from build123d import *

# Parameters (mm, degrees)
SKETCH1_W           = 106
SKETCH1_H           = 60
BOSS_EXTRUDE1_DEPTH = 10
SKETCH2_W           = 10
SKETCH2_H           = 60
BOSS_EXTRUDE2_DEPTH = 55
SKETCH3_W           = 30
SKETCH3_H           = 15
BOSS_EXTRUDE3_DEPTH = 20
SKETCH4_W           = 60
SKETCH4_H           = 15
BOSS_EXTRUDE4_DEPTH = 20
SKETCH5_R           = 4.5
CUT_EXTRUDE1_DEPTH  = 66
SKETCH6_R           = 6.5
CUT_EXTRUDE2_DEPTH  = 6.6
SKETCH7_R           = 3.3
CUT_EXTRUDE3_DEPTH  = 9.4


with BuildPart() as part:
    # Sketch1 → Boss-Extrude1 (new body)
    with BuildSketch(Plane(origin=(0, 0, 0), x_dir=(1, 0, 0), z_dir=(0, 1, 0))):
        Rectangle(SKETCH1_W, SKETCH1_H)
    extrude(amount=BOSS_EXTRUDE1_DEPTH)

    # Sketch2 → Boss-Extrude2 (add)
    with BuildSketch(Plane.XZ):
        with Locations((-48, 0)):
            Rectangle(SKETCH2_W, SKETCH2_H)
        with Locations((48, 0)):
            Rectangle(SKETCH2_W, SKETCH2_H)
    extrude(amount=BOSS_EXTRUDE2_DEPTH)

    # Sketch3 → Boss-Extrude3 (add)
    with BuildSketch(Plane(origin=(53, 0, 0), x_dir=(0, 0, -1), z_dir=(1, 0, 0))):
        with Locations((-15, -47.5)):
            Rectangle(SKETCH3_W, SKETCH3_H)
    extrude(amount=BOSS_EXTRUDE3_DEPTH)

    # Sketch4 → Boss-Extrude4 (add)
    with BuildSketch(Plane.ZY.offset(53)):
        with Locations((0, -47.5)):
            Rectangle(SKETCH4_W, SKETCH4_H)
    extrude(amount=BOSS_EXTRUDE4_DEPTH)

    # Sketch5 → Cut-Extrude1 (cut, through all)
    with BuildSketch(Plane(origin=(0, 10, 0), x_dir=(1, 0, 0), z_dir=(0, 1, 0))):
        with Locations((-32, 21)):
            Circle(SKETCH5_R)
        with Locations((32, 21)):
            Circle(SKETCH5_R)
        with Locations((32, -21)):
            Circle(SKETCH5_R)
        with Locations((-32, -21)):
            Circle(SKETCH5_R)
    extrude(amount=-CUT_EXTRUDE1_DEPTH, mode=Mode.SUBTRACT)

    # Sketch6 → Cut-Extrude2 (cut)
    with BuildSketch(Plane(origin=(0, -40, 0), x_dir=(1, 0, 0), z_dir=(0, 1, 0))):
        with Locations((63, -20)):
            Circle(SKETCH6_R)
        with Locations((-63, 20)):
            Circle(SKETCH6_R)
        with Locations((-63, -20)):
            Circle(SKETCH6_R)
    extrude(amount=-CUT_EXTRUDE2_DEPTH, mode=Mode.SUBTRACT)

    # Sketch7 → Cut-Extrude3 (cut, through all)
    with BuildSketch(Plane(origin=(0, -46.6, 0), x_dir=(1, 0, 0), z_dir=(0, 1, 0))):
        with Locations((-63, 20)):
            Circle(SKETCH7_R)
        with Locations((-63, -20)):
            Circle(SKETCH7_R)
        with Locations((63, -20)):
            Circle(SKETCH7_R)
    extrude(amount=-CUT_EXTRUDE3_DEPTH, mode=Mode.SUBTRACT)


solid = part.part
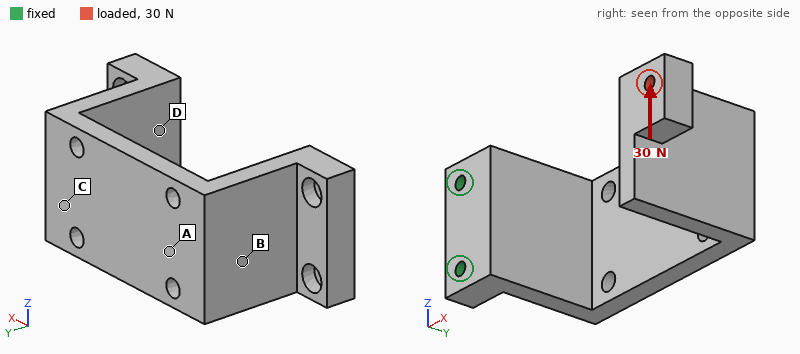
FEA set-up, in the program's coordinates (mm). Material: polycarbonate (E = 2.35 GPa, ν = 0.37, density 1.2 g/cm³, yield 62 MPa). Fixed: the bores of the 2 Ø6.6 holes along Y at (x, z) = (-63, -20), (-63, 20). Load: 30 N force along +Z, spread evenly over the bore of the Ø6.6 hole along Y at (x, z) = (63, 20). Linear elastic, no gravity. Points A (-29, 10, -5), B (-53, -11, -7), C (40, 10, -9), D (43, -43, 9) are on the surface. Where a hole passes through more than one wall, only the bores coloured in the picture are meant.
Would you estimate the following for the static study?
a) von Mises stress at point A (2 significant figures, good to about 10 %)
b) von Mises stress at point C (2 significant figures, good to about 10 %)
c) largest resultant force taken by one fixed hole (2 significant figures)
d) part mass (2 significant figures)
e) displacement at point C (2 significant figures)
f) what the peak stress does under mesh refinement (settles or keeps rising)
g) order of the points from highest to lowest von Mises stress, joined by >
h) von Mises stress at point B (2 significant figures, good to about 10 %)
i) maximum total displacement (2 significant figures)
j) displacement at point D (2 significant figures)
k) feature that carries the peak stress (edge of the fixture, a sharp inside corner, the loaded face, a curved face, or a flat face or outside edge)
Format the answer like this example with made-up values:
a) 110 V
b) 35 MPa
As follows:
a) 1.8 MPa
b) 0.87 MPa
c) 85 N
d) 180 g
e) 0.67 mm
f) keeps rising
g) B > A > C > D
h) 2.5 MPa
i) 1.7 mm
j) 1.3 mm
k) edge of the fixture
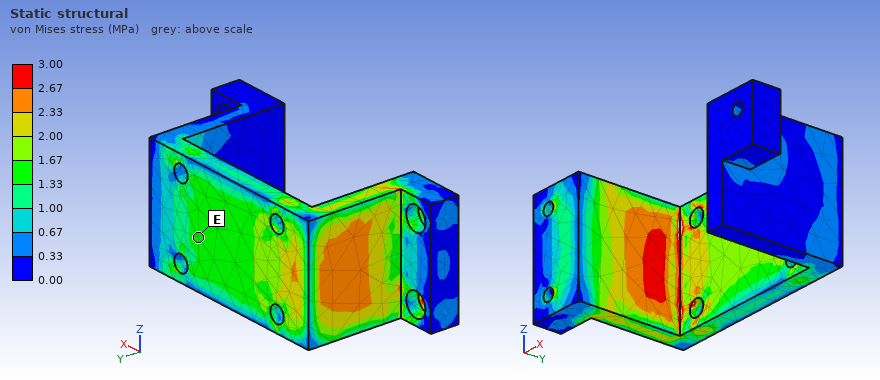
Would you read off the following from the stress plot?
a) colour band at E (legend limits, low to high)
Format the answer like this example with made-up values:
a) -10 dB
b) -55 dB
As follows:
a) 1.33 to 1.67 MPa
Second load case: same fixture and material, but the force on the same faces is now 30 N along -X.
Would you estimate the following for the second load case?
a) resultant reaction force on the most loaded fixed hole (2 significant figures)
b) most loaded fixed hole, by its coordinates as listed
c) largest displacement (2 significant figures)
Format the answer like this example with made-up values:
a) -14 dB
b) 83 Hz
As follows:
a) 28 N
b) (-63, 20)
c) 2.0 mm
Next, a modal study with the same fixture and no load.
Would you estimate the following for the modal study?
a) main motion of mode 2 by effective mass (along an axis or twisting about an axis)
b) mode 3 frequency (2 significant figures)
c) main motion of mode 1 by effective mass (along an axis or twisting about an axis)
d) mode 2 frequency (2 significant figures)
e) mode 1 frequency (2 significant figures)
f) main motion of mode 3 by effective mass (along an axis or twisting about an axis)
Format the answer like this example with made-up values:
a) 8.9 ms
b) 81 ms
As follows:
a) along Z
b) 190 Hz
c) along Y
d) 110 Hz
e) 65 Hz
f) along X
